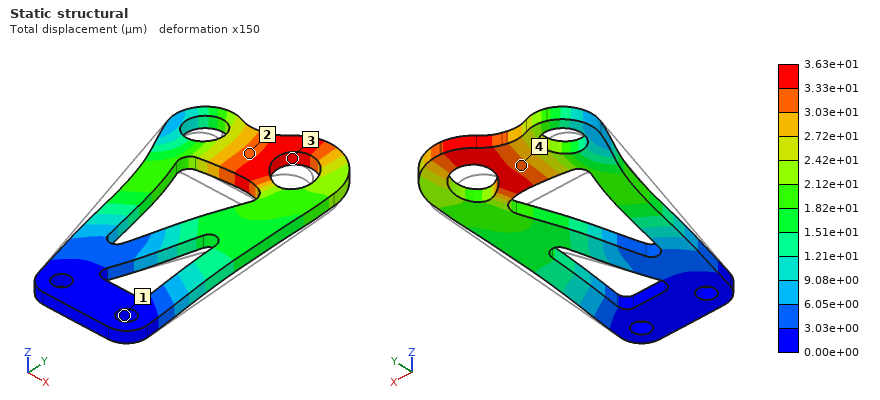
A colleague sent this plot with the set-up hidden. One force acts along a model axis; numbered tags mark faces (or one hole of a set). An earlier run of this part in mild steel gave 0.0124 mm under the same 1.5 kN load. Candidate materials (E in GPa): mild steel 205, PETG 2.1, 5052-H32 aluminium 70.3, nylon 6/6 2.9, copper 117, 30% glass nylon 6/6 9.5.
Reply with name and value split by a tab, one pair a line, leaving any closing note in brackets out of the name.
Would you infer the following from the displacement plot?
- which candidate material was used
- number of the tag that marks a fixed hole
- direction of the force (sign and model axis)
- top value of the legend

which candidate material was used	5052-H32 aluminium
number of the tag that marks a fixed hole	1
direction of the force	+Y
top value of the legend	3.63e+01 µm
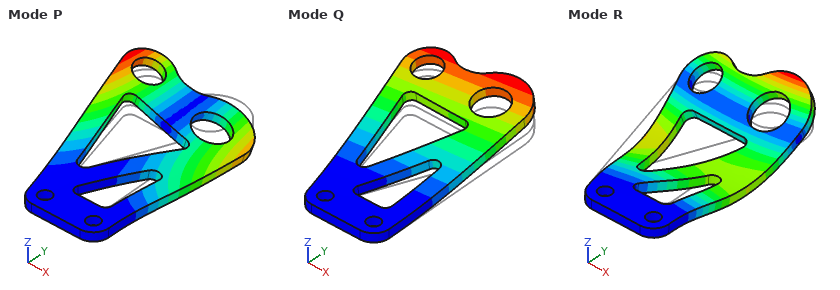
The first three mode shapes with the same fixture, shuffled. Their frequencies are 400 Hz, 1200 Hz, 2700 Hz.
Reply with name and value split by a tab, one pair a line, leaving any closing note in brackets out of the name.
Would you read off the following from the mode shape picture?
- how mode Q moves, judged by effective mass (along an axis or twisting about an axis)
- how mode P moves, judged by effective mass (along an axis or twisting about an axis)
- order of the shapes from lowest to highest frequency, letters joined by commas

how mode Q moves, judged by effective mass	along Z
how mode P moves, judged by effective mass	twisting about Y
order of the shapes from lowest to highest frequency, letters joined by commas	Q, P, R
